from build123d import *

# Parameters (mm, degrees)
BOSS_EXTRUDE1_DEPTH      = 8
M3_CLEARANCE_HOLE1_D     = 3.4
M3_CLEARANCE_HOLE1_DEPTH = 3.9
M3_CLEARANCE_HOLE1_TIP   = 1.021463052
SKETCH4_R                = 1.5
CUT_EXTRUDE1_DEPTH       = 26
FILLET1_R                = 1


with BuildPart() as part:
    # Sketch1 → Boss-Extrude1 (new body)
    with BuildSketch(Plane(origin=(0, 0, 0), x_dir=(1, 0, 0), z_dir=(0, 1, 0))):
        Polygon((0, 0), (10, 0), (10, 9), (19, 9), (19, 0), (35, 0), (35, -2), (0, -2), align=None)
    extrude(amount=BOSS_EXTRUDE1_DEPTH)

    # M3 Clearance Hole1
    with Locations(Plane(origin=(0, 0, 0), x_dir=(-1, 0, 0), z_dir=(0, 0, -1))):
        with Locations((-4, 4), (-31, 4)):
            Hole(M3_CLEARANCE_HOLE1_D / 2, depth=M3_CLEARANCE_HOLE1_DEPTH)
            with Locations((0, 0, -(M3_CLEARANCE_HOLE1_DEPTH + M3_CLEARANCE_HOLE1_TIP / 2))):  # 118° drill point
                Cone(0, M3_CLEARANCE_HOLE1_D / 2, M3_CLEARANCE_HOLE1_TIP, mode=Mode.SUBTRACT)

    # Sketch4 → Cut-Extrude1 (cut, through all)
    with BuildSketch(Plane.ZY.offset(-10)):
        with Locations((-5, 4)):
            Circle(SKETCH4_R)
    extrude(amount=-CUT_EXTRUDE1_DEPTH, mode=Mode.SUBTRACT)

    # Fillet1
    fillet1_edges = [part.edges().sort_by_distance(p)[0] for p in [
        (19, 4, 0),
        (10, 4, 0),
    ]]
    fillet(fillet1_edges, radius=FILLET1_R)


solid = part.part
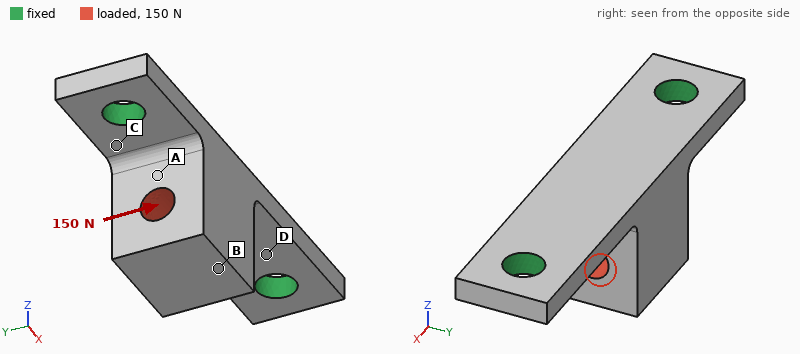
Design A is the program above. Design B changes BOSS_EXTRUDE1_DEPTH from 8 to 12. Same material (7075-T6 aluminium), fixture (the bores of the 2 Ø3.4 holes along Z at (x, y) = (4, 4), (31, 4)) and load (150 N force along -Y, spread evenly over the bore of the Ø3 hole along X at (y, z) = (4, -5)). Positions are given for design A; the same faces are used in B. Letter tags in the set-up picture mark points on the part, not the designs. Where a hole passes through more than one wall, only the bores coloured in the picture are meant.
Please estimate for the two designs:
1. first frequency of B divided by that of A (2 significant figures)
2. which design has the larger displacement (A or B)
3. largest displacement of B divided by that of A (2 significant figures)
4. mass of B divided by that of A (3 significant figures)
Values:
0.88
A
0.72
1.54
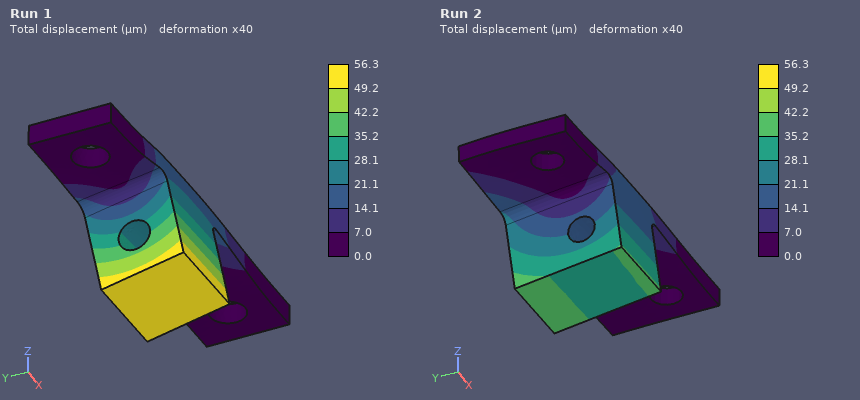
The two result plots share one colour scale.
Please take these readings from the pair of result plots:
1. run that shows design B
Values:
Run 2
